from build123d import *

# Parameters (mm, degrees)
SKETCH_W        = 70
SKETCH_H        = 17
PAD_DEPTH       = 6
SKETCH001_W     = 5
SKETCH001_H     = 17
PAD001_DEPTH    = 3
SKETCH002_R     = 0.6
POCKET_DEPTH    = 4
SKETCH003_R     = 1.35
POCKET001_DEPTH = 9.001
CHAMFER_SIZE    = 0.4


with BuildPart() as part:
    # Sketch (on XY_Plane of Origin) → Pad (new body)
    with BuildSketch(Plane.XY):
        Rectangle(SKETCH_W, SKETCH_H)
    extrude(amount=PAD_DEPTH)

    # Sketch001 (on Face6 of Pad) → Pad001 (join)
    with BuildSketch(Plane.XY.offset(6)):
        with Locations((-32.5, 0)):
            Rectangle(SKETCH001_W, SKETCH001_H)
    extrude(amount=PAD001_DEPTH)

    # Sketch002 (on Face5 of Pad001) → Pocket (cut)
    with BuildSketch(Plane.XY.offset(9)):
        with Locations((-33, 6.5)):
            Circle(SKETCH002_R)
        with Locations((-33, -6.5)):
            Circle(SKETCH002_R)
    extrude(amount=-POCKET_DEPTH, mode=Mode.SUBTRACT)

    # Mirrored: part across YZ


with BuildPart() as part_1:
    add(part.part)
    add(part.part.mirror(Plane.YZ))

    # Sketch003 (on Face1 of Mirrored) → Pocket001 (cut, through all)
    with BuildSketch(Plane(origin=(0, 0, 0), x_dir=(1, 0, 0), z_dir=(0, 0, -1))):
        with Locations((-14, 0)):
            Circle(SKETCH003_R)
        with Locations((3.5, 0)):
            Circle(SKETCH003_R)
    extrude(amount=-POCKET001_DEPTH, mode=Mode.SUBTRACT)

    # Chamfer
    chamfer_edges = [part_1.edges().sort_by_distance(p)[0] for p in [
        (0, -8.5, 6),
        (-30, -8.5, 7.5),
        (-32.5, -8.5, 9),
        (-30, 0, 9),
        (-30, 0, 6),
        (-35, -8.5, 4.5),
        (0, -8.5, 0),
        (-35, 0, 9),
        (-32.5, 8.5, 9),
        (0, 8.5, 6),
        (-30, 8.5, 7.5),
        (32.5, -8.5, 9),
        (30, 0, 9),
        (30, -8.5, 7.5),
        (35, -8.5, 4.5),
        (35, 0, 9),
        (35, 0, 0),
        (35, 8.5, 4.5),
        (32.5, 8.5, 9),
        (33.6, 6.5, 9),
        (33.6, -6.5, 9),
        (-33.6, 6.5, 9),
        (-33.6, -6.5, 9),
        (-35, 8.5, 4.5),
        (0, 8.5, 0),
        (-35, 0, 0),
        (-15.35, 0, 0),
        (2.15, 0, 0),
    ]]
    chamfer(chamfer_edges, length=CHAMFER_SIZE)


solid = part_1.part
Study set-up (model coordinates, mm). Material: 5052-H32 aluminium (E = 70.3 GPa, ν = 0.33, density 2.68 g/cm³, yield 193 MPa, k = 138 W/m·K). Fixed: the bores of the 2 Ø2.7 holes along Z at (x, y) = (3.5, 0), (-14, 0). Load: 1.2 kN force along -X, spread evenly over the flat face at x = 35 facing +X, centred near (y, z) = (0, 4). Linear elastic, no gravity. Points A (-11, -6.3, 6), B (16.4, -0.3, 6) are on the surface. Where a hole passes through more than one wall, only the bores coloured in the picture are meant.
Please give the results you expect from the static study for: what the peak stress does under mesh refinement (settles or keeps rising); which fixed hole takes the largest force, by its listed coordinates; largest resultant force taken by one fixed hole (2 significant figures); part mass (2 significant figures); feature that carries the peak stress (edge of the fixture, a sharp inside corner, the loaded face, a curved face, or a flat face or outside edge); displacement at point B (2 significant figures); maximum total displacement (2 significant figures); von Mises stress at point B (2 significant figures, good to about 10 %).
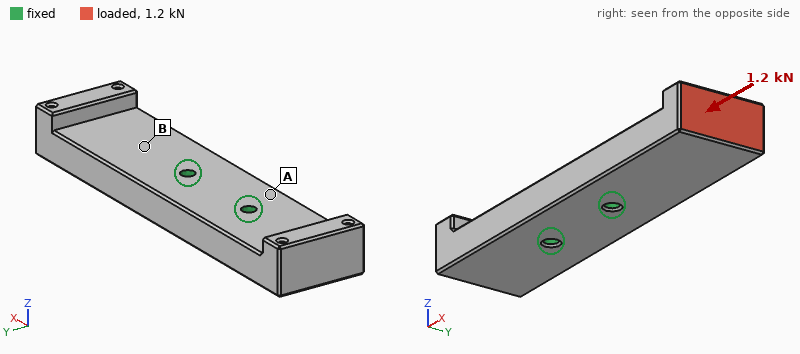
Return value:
keeps rising
(3.5, 0)
980 N
20 g
edge of the fixture
11 µm
48 µm
30 MPa
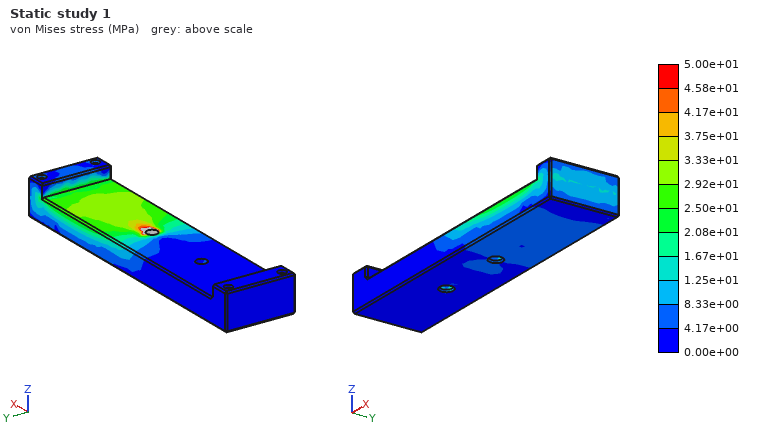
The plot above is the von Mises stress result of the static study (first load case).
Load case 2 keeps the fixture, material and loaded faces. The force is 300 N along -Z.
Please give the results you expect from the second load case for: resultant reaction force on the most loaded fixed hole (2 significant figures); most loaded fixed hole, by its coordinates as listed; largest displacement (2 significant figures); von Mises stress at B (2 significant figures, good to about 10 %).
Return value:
500 N
(3.5, 0)
0.17 mm
53 MPa
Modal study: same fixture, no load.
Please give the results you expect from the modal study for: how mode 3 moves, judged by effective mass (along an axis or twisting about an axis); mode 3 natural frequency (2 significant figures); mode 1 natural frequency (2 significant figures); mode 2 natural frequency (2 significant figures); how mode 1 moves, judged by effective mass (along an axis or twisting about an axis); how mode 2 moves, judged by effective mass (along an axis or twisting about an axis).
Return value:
along Z
8400 Hz
4100 Hz
7900 Hz
along Z
along Y
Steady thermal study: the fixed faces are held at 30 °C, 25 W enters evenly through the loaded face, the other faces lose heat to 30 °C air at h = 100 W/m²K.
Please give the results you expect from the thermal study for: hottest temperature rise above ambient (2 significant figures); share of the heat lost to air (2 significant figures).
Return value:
51 K
18 %
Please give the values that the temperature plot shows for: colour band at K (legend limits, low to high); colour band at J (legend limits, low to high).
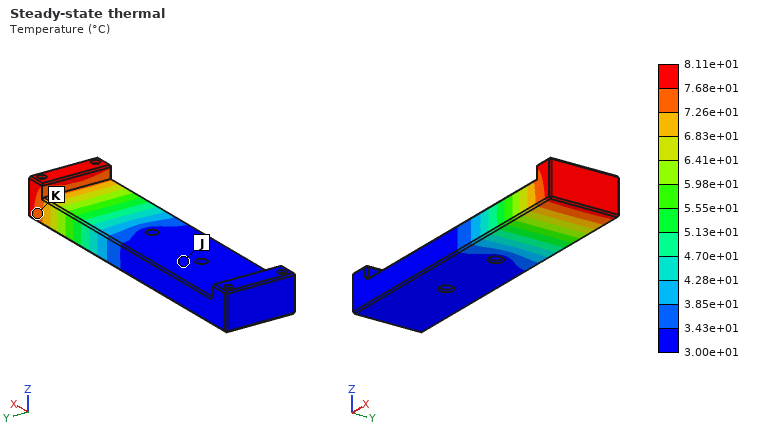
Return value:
7.26e+01 to 7.68e+01 °C
3.00e+01 to 3.43e+01 °C
